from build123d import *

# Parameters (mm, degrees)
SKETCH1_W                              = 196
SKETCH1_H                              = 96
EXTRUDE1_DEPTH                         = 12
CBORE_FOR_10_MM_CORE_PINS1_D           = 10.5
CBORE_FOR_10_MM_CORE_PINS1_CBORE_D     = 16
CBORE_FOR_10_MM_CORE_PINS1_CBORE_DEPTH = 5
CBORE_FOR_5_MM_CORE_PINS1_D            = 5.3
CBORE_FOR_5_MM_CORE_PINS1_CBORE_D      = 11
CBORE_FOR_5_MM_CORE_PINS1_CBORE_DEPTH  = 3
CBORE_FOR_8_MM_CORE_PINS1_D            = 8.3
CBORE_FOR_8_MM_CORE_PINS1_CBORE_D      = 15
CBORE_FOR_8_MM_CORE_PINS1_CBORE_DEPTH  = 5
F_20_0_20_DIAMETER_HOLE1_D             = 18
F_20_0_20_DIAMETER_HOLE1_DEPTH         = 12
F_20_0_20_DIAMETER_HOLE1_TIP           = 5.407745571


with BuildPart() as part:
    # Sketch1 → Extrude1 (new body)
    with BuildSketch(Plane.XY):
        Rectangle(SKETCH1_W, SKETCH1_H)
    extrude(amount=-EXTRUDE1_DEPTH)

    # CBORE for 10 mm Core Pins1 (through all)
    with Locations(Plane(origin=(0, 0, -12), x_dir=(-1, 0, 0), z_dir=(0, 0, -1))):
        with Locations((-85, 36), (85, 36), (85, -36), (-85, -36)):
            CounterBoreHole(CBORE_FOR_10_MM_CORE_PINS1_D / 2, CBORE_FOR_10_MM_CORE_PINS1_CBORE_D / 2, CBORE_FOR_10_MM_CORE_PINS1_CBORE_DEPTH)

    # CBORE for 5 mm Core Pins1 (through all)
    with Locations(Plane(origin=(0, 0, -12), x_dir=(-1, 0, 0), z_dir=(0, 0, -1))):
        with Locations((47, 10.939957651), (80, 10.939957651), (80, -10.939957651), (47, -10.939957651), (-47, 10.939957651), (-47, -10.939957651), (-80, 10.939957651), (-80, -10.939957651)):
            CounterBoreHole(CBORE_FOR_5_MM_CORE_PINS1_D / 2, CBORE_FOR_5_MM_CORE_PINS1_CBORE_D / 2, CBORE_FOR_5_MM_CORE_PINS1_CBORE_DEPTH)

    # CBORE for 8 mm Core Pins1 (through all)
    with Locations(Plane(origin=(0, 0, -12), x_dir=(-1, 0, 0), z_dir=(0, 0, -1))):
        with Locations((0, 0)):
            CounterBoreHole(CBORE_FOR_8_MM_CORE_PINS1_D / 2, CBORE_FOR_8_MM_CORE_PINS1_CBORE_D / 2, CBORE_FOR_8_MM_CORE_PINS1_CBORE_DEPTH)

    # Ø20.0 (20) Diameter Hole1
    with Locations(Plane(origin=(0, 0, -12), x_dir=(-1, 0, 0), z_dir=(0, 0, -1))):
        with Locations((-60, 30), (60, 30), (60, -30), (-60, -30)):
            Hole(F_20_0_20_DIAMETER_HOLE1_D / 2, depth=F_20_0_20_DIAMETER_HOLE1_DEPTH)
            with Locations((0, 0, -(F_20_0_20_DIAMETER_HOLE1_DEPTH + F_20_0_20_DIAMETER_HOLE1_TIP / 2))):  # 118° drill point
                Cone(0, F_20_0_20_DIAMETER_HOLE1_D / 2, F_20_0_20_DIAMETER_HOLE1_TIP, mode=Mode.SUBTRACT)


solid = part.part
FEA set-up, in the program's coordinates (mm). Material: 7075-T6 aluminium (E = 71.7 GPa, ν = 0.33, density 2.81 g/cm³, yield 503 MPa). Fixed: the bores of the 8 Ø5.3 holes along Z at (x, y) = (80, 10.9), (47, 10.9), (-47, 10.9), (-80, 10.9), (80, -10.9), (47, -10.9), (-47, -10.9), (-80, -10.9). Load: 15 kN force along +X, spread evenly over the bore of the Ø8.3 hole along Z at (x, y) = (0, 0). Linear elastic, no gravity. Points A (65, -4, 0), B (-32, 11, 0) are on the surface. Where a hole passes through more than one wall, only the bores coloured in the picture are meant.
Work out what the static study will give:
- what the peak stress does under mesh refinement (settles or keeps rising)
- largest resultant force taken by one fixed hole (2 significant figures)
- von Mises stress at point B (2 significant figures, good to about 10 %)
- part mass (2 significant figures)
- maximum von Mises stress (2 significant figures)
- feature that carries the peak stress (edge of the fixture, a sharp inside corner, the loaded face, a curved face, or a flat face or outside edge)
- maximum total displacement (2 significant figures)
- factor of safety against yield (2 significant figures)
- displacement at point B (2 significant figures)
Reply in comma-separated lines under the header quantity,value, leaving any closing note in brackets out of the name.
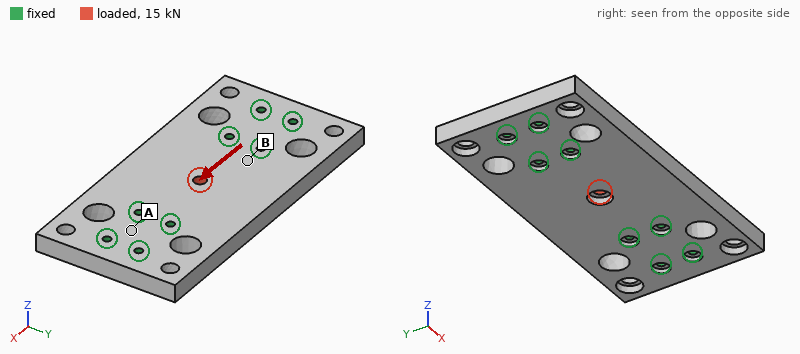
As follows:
quantity,value
what the peak stress does under mesh refinement,settles
largest resultant force taken by one fixed hole,3.2 kN
von Mises stress at point B,18 MPa
part mass,570 g
maximum von Mises stress,140 MPa
feature that carries the peak stress,the loaded face
maximum total displacement,19 µm
factor of safety against yield,3.6
displacement at point B,3.6 µm
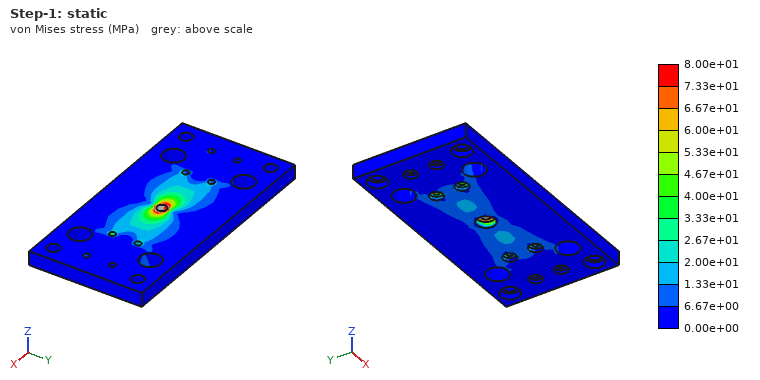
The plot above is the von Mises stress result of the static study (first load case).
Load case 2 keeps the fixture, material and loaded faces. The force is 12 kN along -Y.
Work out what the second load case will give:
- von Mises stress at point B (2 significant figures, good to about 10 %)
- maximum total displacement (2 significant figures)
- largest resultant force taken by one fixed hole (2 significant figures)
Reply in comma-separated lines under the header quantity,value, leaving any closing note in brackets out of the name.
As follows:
quantity,value
von Mises stress at point B,15 MPa
maximum total displacement,23 µm
largest resultant force taken by one fixed hole,3.2 kN
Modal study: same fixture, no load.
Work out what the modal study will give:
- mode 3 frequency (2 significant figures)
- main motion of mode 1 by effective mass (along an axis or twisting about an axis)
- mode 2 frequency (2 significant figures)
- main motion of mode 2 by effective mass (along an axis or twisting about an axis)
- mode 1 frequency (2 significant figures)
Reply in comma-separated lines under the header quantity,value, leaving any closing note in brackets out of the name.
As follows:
quantity,value
mode 3 frequency,5900 Hz
main motion of mode 1 by effective mass,twisting about X
mode 2 frequency,4000 Hz
main motion of mode 2 by effective mass,along Z
mode 1 frequency,3700 Hz
